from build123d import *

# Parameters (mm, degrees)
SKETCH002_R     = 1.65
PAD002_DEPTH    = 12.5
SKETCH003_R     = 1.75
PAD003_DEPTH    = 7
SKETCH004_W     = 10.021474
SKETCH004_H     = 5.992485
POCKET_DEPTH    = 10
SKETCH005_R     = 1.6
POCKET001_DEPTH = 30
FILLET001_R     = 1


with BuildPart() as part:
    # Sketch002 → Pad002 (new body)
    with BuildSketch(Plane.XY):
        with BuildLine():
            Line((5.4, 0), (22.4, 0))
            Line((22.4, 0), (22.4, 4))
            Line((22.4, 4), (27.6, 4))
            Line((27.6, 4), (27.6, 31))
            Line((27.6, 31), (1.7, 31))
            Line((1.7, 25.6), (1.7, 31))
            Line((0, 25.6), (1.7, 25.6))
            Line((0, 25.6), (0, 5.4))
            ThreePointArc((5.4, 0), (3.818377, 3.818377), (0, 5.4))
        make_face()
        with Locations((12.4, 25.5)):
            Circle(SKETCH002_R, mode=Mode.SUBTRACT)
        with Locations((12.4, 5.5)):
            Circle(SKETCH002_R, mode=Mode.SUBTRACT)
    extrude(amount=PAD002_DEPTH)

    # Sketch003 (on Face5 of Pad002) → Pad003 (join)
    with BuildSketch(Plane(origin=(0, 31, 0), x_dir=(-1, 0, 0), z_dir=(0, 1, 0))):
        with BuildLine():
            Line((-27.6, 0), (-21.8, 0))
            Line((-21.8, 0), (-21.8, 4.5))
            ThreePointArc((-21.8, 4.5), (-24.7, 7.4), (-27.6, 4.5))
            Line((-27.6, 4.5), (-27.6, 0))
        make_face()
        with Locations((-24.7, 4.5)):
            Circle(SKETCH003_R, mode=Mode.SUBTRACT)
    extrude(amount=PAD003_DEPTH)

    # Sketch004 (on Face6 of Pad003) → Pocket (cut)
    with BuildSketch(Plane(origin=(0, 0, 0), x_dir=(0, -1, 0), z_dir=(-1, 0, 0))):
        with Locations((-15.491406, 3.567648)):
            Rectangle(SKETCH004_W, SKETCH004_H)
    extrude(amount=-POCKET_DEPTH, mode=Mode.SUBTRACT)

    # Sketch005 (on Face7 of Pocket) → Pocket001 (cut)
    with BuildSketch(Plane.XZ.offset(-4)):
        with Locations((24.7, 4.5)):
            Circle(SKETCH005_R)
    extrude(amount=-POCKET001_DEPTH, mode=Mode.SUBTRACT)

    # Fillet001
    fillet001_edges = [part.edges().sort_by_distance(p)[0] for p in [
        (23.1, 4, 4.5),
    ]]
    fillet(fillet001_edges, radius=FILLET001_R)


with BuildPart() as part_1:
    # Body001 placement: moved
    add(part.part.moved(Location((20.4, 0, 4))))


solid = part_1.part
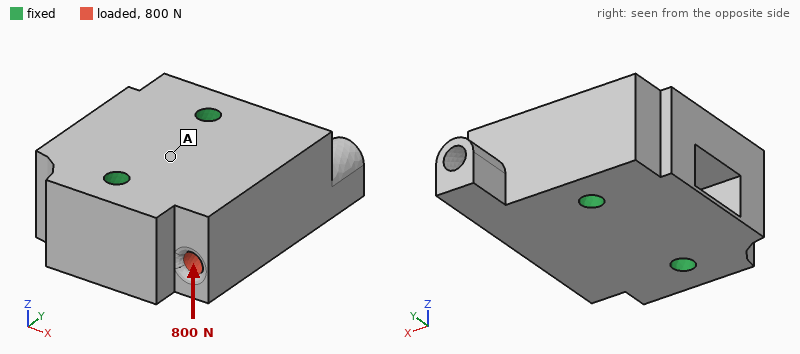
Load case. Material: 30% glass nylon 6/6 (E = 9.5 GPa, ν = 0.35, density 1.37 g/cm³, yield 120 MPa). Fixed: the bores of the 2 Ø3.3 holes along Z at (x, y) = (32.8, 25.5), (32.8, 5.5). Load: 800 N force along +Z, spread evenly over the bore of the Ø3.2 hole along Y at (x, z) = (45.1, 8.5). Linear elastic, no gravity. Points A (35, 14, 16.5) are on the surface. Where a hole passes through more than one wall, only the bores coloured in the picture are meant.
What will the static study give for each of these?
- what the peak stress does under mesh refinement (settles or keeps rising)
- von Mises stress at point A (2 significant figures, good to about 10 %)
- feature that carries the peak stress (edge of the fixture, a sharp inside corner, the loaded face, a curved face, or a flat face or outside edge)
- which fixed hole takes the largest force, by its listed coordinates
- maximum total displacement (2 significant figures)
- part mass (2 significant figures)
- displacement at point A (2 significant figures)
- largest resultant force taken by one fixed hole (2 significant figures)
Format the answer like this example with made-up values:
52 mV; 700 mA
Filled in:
keeps rising; 5.1 MPa; edge of the fixture; (32.8, 25.5); 38 µm; 13 g; 9.9 µm; 470 N
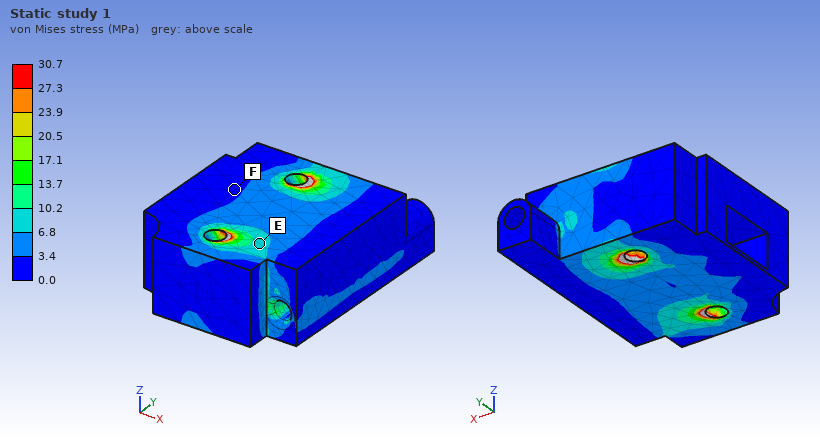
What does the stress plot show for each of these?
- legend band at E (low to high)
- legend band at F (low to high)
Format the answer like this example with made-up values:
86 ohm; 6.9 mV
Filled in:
6.8 to 10.2 MPa; 0.0 to 3.4 MPa
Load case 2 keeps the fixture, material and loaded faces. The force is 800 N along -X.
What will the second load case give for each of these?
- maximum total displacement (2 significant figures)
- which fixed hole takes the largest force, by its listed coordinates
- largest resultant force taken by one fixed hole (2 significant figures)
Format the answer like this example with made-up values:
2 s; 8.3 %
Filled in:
9.2 µm; (32.8, 25.5); 500 N
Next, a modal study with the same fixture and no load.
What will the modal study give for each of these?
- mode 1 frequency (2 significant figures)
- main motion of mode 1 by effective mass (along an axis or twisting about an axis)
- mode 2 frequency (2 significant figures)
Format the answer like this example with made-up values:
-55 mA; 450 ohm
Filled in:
14 kHz; along Z; 18 kHz
